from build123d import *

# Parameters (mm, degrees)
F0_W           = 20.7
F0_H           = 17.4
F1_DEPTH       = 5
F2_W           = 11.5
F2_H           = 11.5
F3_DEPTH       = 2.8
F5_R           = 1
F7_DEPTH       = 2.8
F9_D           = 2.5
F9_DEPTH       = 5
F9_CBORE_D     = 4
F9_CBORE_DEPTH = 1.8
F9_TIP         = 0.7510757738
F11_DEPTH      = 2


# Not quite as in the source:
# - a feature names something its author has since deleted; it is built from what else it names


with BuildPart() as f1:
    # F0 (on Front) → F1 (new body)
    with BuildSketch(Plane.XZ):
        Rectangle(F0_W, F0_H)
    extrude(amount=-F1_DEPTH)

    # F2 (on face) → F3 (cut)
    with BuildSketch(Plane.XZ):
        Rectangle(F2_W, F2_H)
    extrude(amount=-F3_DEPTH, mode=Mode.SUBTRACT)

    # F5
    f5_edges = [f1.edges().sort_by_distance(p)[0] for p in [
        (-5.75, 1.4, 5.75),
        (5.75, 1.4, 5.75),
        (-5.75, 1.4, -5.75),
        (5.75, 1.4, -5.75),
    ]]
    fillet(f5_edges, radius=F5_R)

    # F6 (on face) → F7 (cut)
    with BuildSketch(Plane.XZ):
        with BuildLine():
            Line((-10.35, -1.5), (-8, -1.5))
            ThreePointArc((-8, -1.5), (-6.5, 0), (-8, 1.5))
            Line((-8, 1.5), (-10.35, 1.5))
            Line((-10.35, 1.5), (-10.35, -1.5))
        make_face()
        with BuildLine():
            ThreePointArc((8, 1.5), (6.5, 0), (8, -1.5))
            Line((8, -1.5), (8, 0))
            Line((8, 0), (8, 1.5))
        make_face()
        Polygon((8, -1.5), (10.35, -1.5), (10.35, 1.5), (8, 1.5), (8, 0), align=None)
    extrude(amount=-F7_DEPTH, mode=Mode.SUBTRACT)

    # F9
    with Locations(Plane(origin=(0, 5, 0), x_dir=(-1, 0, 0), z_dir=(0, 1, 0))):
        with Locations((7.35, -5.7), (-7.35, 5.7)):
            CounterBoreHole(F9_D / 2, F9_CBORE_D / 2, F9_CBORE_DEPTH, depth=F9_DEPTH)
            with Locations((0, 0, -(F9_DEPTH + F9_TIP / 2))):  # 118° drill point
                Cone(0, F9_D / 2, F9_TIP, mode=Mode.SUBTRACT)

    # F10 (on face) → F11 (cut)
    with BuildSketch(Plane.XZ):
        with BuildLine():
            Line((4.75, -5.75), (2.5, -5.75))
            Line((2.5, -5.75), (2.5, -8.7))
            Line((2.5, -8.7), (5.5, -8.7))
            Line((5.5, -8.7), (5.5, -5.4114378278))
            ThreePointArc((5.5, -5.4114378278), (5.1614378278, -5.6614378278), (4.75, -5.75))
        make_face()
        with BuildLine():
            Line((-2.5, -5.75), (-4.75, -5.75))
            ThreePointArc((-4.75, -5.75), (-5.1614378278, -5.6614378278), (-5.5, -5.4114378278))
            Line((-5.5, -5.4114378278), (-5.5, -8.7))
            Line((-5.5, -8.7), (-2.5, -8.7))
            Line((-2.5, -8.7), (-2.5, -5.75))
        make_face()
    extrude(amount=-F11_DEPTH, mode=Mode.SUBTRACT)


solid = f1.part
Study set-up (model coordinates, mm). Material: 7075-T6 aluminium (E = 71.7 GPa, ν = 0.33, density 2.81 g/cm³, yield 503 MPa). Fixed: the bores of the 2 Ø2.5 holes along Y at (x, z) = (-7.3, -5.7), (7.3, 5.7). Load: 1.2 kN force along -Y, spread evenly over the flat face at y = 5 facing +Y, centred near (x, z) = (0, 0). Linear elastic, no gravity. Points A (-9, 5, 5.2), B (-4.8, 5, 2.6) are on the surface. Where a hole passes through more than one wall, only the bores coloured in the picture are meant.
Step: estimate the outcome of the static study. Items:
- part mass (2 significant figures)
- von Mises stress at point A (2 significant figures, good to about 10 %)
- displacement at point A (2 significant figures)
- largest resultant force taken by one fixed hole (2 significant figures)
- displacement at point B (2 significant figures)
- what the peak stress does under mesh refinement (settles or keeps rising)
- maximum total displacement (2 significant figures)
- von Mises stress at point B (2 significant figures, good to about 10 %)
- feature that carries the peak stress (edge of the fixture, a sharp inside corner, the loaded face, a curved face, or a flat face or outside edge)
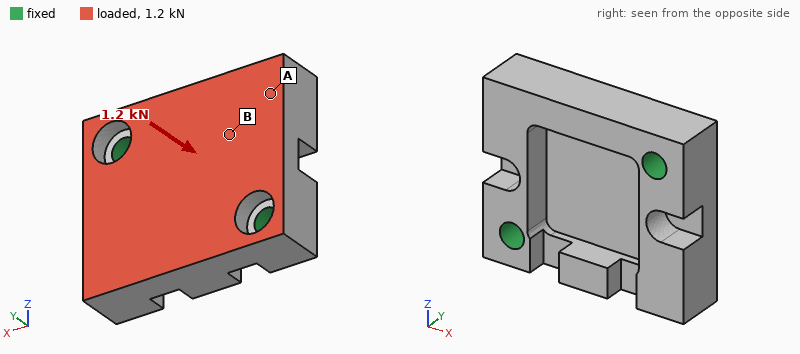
3.5 g
17 MPa
22 µm
810 N
14 µm
keeps rising
49 µm
54 MPa
edge of the fixture
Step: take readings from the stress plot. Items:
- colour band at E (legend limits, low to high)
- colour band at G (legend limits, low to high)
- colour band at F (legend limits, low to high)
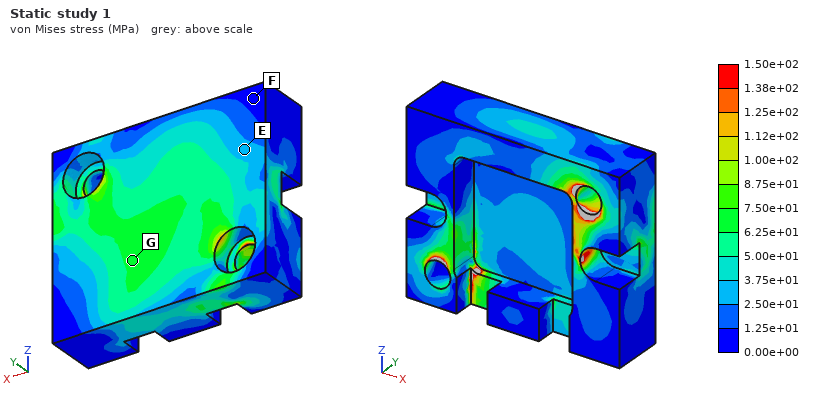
2.50e+01 to 3.75e+01 MPa
6.25e+01 to 7.50e+01 MPa
0.00e+00 to 1.25e+01 MPa
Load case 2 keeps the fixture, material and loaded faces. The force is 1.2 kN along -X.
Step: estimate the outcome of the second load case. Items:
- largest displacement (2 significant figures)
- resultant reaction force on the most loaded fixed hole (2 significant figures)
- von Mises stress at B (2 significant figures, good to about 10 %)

26 µm
630 N
16 MPa
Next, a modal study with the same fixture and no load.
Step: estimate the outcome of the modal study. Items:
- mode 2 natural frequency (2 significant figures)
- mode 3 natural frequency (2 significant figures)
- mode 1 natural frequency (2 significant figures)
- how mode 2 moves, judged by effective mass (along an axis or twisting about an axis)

19 kHz
37 kHz
14 kHz
along Y
